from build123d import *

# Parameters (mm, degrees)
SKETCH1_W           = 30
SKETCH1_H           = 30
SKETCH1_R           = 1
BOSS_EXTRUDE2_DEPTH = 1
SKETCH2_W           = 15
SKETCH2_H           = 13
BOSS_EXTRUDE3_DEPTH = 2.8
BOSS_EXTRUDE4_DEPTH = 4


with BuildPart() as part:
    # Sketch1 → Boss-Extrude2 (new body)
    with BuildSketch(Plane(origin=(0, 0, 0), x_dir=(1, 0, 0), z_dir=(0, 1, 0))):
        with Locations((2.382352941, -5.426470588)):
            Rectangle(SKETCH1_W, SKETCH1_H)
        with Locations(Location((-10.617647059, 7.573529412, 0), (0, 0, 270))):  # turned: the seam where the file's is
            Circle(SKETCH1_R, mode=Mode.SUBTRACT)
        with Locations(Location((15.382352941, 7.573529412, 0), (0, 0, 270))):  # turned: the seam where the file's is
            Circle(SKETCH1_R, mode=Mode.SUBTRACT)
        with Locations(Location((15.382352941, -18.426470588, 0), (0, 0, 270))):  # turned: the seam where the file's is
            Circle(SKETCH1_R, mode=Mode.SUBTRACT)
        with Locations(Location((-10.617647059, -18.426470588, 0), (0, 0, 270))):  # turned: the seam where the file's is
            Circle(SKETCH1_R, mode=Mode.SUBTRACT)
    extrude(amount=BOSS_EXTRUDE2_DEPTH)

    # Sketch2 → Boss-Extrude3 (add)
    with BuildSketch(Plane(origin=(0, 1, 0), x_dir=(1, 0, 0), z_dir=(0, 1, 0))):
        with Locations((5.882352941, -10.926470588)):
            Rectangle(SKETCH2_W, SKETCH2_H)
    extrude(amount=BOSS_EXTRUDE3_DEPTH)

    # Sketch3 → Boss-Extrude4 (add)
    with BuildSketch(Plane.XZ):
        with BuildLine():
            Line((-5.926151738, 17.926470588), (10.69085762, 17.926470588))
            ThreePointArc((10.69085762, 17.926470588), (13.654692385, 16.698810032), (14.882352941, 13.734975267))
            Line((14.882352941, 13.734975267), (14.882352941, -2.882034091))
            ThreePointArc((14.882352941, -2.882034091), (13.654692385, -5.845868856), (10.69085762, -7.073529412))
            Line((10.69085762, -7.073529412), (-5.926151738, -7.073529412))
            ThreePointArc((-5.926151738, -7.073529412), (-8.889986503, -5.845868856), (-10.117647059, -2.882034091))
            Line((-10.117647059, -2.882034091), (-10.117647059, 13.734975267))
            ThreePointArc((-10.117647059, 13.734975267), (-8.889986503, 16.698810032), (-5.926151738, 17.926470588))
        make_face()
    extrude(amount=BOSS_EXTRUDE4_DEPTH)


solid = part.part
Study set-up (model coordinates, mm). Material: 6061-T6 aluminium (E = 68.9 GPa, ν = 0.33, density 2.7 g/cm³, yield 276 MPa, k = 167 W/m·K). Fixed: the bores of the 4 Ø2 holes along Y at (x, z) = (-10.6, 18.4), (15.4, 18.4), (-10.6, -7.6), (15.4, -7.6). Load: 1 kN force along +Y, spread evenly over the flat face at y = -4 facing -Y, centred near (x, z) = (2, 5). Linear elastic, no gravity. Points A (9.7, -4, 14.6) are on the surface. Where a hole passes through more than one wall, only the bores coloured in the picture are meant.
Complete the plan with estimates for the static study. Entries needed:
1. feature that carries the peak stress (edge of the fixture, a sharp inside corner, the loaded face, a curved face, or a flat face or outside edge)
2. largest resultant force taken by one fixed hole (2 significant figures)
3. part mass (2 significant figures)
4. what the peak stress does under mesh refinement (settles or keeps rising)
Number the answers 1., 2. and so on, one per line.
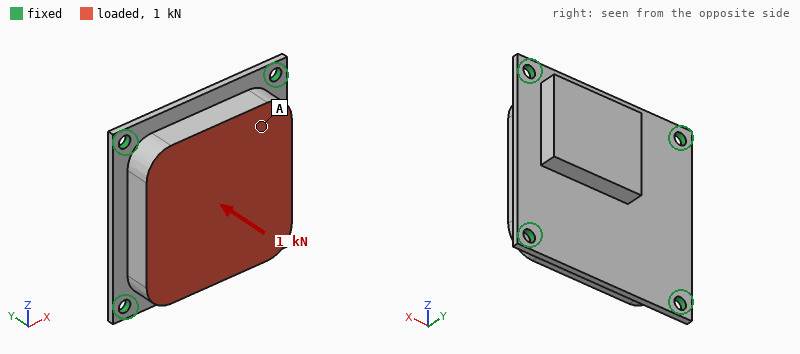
1. edge of the fixture
2. 330 N
3. 10 g
4. keeps rising
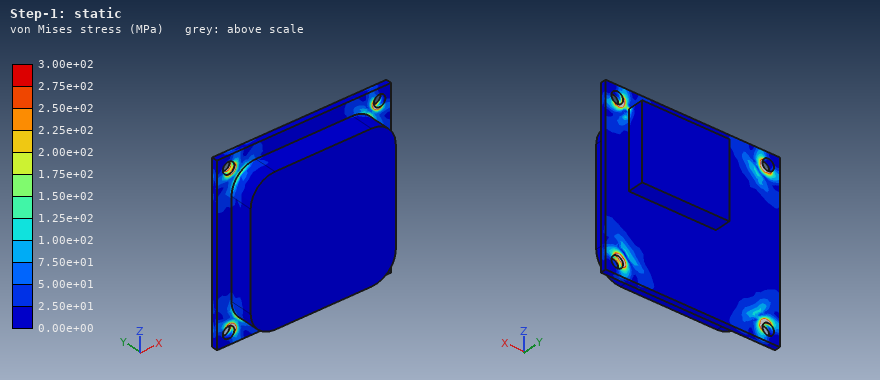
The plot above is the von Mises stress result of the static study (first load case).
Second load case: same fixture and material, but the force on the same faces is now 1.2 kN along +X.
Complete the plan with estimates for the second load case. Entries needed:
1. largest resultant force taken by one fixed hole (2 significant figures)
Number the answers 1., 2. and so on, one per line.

1. 360 N
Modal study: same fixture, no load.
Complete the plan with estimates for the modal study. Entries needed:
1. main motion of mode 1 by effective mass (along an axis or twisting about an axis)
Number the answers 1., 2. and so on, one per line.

1. along Y
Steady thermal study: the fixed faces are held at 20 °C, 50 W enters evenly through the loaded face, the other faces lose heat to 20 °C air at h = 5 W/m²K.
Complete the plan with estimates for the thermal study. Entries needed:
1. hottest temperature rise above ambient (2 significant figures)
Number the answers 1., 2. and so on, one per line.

1. 45 K
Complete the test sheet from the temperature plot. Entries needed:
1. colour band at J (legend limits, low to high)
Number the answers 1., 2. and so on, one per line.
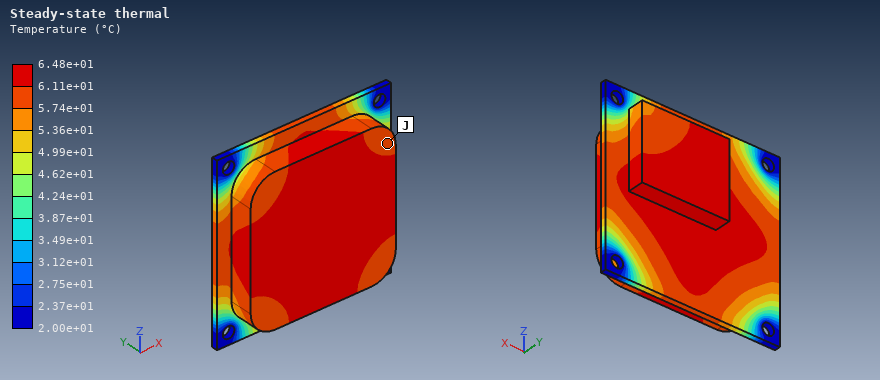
1. 5.74e+01 to 6.11e+01 °C
